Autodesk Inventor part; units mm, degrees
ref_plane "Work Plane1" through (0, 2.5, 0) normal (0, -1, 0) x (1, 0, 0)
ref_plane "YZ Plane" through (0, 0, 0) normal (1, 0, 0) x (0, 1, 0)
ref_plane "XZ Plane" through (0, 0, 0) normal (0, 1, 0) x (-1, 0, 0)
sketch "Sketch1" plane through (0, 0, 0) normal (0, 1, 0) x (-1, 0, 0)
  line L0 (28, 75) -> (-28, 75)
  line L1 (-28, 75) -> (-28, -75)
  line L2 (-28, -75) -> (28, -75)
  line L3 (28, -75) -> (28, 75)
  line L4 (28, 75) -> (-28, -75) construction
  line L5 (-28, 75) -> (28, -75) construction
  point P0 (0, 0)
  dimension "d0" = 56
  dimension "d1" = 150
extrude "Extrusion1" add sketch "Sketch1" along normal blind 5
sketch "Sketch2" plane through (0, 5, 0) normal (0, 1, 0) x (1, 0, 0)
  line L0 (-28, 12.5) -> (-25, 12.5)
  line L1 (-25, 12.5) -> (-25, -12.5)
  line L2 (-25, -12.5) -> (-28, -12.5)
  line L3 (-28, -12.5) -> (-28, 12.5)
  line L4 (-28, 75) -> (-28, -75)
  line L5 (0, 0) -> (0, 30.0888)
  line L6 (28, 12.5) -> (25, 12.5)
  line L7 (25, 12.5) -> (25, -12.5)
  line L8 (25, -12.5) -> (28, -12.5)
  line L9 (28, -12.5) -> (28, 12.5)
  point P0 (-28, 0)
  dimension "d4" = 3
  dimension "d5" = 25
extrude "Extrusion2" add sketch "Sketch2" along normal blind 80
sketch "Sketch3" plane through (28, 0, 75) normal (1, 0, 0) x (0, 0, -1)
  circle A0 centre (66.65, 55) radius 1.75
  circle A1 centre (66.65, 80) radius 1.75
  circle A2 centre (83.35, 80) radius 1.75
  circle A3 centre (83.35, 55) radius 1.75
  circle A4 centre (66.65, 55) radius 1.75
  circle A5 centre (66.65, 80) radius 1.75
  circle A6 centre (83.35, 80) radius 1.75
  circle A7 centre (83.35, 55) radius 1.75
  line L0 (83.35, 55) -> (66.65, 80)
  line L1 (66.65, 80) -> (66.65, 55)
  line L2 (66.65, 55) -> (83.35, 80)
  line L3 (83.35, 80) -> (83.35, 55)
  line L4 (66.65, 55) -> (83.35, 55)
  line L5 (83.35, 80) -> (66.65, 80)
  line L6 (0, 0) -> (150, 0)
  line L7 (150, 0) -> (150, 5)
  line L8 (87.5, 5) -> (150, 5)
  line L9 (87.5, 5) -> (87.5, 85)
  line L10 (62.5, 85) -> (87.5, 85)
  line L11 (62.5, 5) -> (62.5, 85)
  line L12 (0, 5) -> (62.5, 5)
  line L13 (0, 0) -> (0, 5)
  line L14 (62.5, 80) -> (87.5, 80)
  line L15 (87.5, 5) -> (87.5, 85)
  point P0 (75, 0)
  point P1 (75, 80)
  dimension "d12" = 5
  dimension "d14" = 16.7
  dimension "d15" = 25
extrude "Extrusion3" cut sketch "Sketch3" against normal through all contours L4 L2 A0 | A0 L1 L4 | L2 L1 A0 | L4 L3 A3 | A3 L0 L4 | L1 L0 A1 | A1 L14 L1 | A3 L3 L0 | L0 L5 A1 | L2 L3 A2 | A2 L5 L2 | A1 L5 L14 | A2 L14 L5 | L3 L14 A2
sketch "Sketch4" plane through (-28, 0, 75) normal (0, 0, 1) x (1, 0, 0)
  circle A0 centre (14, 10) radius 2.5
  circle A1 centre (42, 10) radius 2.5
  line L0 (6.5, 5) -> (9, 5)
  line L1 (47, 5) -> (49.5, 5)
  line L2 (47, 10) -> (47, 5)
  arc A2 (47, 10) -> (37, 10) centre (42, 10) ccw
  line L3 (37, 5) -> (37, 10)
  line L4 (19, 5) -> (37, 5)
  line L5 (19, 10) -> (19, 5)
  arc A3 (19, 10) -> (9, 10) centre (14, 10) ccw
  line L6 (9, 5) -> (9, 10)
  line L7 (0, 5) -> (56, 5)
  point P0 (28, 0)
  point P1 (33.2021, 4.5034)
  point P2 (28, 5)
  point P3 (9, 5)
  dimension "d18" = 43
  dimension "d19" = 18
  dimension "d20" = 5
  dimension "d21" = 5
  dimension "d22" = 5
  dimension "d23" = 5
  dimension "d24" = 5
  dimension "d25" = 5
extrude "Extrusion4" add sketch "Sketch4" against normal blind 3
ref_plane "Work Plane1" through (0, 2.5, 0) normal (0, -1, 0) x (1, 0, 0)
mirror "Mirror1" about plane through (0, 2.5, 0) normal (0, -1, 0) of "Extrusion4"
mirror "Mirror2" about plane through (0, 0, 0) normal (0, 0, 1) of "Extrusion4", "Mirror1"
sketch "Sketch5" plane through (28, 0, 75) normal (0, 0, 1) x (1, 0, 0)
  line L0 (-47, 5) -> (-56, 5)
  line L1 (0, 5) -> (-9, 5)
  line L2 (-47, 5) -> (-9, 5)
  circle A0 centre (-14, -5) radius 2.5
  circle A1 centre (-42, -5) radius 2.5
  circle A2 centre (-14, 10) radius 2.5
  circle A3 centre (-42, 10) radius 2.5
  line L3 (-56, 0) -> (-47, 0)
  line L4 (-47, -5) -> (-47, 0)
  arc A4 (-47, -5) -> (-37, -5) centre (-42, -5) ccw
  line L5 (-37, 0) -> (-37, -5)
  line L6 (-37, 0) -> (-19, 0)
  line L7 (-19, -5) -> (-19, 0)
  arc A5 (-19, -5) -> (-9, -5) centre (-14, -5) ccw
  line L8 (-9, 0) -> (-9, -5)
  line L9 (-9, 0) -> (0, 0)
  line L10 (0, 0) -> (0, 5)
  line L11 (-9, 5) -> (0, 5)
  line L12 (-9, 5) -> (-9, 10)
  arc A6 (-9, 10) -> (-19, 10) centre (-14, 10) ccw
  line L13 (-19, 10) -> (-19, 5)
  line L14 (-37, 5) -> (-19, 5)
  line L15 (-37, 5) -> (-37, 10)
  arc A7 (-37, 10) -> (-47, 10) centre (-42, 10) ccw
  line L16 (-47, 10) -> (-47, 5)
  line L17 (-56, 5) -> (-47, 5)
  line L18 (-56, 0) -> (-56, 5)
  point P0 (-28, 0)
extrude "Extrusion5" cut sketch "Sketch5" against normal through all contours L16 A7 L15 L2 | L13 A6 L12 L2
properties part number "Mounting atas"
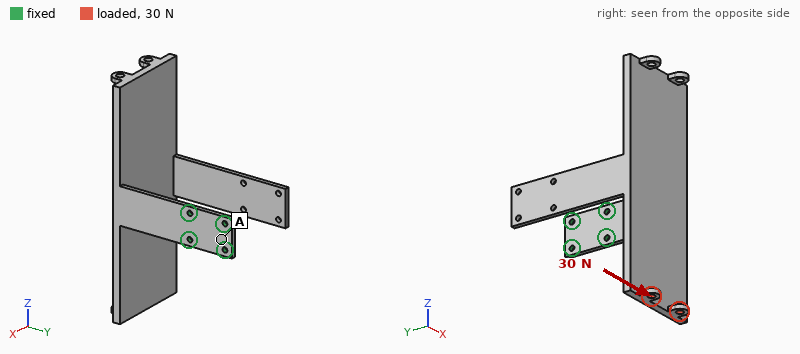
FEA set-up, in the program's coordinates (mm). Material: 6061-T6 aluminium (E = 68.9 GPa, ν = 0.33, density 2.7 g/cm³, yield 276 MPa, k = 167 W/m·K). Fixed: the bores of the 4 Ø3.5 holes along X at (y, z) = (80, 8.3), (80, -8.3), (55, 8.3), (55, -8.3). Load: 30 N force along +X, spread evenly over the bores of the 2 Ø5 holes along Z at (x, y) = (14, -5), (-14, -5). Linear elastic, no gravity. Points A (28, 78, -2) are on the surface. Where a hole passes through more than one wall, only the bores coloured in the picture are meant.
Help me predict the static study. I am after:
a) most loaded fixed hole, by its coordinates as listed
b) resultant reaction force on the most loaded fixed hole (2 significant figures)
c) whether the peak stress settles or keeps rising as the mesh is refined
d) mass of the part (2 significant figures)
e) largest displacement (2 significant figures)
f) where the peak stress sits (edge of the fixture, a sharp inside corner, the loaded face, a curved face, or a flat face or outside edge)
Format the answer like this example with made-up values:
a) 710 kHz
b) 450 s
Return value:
a) (55, -8.3)
b) 140 N
c) keeps rising
d) 150 g
e) 2.0 mm
f) edge of the fixture
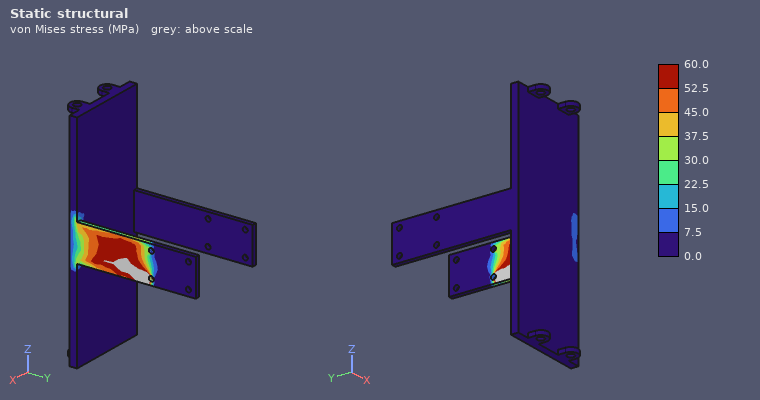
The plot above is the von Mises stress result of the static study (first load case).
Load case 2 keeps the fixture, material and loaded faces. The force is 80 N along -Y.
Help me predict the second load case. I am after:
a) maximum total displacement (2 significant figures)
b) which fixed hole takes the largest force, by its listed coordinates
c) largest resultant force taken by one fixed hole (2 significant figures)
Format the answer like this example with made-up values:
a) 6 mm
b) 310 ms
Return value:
a) 2.2 mm
b) (55, -8.3)
c) 350 N
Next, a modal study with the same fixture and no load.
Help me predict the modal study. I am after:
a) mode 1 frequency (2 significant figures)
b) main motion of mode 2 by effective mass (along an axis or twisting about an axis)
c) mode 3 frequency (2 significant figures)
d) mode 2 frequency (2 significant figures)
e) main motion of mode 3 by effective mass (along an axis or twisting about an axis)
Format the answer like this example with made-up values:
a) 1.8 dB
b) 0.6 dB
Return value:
a) 86 Hz
b) along Z
c) 260 Hz
d) 96 Hz
e) along X
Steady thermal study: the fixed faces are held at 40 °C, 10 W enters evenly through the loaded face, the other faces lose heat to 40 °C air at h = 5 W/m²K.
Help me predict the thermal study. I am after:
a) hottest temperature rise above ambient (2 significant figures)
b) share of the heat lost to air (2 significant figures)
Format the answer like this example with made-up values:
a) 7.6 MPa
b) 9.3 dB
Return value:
a) 52 K
b) 38 %
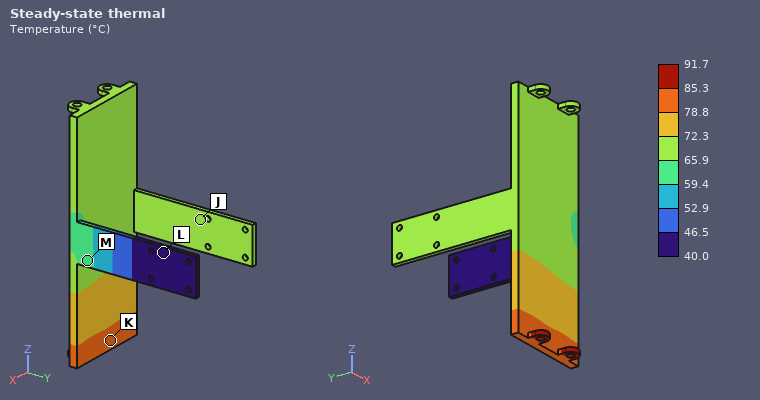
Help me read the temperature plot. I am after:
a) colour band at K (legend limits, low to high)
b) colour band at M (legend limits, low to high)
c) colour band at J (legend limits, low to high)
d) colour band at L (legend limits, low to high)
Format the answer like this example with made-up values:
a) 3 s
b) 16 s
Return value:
a) 78.8 to 85.3 °C
b) 59.4 to 65.9 °C
c) 65.9 to 72.3 °C
d) 40.0 to 46.5 °C
